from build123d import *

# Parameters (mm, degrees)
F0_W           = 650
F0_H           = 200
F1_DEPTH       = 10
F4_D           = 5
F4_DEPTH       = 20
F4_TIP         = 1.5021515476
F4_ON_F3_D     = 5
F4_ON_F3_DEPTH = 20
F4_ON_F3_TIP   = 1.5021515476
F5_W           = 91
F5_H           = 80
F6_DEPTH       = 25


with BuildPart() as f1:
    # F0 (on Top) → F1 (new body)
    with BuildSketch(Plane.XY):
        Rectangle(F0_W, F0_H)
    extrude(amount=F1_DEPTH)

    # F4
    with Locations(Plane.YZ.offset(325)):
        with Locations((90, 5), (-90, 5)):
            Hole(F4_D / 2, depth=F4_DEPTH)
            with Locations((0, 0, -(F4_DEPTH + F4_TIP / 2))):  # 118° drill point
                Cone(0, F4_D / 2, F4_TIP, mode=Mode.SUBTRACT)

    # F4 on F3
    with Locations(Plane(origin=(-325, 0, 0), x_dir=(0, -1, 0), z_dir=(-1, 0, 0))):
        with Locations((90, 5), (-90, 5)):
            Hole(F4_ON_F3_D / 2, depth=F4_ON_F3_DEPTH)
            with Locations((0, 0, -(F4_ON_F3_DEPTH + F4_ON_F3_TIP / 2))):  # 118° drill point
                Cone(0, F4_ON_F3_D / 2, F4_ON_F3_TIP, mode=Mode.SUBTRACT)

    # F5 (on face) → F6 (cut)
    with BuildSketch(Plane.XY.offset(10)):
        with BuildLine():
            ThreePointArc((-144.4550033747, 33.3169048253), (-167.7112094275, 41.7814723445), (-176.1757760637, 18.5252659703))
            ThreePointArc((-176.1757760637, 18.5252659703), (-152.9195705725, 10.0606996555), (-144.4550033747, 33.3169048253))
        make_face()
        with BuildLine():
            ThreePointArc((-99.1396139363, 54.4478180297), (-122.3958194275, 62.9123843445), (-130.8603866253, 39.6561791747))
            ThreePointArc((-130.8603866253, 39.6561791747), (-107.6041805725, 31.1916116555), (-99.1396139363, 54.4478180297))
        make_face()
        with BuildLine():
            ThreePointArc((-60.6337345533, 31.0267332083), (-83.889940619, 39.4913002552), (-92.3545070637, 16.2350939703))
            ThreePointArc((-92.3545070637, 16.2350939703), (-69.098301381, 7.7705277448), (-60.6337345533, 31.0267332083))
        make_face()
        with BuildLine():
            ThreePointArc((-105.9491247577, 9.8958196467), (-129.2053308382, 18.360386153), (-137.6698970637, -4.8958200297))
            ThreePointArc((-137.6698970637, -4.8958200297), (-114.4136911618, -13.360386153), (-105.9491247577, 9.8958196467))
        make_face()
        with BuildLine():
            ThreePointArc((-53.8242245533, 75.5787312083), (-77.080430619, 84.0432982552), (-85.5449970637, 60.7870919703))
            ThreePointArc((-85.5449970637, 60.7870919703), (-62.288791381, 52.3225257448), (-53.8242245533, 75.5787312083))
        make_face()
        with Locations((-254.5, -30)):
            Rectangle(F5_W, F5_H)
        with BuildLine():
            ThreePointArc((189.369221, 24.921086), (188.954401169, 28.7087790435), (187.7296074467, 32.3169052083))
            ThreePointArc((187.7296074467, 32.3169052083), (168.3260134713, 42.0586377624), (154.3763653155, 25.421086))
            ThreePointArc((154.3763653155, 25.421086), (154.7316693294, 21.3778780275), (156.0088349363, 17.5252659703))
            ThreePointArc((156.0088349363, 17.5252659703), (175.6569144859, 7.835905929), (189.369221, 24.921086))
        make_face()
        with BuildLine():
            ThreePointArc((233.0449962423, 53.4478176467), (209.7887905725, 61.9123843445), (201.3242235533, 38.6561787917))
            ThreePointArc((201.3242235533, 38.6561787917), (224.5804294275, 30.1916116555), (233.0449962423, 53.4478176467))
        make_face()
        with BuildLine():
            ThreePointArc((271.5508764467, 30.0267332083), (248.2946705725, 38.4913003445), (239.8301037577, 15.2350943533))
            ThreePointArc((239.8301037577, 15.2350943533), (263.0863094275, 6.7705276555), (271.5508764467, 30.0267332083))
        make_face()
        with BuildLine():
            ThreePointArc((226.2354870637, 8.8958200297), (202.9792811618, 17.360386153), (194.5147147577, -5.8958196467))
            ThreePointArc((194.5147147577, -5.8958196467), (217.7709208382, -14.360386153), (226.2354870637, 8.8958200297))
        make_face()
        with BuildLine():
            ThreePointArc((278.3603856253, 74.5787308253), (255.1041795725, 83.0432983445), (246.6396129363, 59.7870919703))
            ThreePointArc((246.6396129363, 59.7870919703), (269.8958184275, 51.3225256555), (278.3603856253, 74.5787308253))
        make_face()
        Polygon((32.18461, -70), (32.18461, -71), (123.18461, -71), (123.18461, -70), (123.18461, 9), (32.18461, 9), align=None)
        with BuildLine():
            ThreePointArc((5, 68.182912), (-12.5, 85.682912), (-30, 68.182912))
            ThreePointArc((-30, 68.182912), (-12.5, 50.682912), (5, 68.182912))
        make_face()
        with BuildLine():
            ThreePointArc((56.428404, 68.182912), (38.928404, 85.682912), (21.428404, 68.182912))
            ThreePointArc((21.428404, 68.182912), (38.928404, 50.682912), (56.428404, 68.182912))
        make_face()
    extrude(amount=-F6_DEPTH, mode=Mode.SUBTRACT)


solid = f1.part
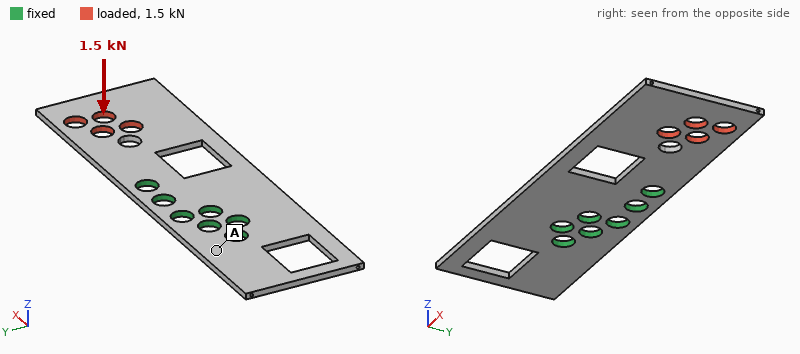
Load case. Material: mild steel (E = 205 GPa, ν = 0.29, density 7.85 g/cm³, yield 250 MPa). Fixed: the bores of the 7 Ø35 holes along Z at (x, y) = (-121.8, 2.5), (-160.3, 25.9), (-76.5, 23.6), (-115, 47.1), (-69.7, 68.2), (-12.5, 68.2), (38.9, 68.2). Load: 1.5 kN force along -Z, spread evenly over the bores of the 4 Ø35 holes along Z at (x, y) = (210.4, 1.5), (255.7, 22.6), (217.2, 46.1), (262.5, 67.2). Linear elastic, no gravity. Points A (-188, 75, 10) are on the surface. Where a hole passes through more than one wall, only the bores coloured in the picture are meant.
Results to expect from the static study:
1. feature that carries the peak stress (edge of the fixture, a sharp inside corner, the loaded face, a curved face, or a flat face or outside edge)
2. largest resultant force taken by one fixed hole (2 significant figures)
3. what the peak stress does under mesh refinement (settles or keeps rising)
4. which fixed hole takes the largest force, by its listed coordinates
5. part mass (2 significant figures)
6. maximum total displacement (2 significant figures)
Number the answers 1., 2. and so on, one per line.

1. edge of the fixture
2. 2.2 kN
3. keeps rising
4. (38.9, 68.2)
5. 8.1 kg
6. 2.9 mm
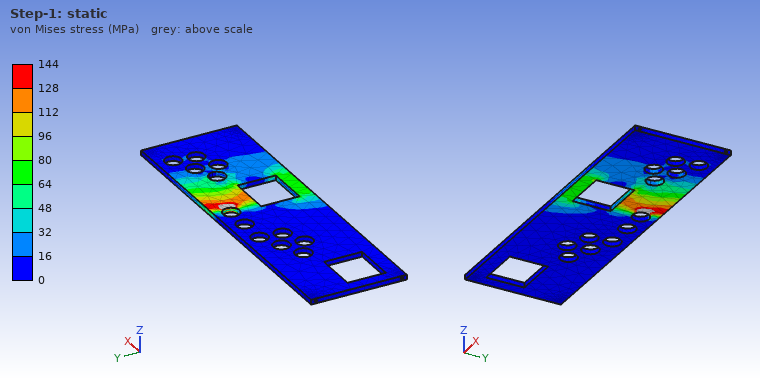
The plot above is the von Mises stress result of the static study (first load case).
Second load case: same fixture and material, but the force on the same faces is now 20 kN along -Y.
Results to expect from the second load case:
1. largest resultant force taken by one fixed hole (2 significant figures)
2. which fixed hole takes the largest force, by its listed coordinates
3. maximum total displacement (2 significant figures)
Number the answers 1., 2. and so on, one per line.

1. 36 kN
2. (38.9, 68.2)
3. 0.23 mm
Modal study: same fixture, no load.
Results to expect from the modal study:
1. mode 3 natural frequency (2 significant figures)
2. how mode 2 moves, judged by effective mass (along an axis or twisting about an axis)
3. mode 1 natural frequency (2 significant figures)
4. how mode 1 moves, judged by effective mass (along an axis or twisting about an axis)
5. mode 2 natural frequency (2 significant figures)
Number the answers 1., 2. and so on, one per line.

1. 300 Hz
2. twisting about X
3. 83 Hz
4. along Z
5. 250 Hz
